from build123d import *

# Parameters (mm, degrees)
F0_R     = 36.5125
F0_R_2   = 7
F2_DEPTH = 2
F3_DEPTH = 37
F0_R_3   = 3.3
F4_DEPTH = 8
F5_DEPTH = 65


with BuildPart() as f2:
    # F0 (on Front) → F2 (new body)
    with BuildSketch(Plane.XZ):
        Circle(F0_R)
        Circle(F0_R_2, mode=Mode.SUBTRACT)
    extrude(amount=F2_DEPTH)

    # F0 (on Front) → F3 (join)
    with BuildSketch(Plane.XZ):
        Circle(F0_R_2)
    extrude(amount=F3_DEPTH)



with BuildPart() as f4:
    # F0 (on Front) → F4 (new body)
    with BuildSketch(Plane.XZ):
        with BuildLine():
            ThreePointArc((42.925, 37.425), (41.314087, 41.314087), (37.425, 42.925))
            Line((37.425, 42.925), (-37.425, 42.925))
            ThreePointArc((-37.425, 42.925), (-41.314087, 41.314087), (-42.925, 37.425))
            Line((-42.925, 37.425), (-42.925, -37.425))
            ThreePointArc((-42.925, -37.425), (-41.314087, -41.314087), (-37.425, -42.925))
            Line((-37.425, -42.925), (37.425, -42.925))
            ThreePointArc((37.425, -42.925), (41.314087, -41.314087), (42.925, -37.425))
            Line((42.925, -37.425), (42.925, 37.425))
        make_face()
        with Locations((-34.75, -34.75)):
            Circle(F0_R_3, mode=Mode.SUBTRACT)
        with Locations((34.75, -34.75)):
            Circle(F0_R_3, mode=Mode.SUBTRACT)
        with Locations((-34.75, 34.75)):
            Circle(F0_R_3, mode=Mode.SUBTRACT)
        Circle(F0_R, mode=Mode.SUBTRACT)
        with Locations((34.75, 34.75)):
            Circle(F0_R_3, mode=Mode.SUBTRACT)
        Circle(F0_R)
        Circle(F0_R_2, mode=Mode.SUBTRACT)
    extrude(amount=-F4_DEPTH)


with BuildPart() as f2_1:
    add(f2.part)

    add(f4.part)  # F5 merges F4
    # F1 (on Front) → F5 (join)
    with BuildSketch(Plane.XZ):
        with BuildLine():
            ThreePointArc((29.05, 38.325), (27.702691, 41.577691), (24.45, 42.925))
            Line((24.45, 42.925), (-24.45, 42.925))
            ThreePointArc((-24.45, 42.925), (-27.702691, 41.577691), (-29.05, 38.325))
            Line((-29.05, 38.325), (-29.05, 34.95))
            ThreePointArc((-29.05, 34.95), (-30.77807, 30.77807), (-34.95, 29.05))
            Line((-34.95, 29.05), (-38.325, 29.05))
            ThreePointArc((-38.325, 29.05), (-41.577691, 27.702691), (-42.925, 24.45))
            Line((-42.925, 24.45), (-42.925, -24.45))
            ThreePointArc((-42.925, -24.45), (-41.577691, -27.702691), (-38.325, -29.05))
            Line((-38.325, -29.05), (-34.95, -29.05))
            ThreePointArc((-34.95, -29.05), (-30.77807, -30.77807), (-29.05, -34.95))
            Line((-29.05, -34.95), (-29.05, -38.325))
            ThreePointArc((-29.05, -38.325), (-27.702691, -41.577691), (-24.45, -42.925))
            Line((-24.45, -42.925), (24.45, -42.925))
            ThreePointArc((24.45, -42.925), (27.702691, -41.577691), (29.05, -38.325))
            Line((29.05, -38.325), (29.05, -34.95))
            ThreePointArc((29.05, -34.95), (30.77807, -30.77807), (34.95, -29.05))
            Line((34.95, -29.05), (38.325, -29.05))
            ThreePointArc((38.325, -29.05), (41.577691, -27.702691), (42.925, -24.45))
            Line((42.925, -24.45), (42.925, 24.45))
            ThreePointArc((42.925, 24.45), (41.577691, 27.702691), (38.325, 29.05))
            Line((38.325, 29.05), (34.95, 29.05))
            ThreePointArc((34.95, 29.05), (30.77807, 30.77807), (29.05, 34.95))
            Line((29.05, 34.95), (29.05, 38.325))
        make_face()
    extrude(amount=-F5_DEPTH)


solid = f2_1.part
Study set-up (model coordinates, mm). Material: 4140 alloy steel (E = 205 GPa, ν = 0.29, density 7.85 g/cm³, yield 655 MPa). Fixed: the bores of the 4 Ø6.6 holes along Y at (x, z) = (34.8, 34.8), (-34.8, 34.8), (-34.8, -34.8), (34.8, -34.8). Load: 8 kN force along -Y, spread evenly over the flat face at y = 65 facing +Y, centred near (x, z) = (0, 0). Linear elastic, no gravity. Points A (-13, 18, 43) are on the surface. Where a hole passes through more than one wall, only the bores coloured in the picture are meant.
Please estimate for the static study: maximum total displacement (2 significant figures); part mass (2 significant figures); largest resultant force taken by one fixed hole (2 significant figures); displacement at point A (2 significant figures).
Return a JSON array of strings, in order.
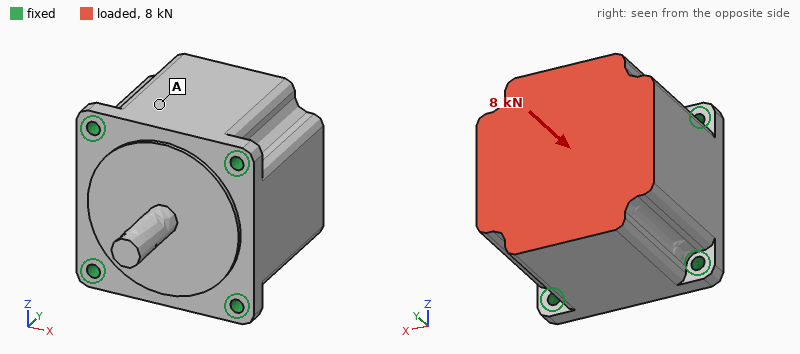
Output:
["1.9 µm", "3.5 kg", "2.1 kN", "1.6 µm"]
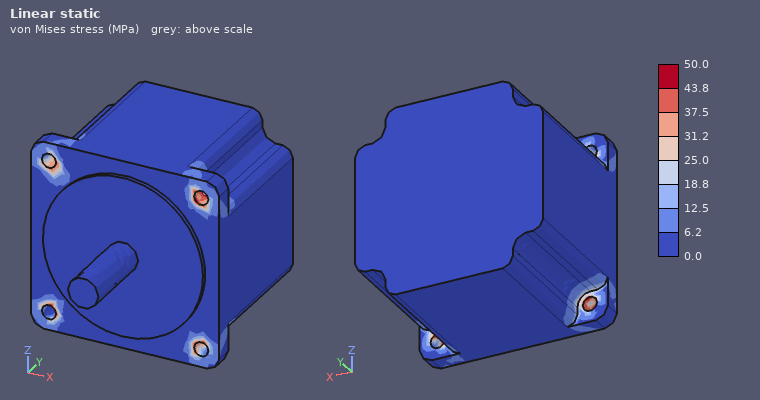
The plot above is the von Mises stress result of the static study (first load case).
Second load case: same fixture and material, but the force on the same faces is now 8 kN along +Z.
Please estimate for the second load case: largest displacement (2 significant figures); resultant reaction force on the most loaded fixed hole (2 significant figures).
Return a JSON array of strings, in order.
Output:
["8.3 µm", "4.3 kN"]
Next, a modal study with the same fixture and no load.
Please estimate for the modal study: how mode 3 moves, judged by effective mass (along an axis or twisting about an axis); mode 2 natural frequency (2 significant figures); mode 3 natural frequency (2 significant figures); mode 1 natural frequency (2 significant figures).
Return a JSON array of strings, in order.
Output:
["along Y", "4500 Hz", "6000 Hz", "4500 Hz"]
